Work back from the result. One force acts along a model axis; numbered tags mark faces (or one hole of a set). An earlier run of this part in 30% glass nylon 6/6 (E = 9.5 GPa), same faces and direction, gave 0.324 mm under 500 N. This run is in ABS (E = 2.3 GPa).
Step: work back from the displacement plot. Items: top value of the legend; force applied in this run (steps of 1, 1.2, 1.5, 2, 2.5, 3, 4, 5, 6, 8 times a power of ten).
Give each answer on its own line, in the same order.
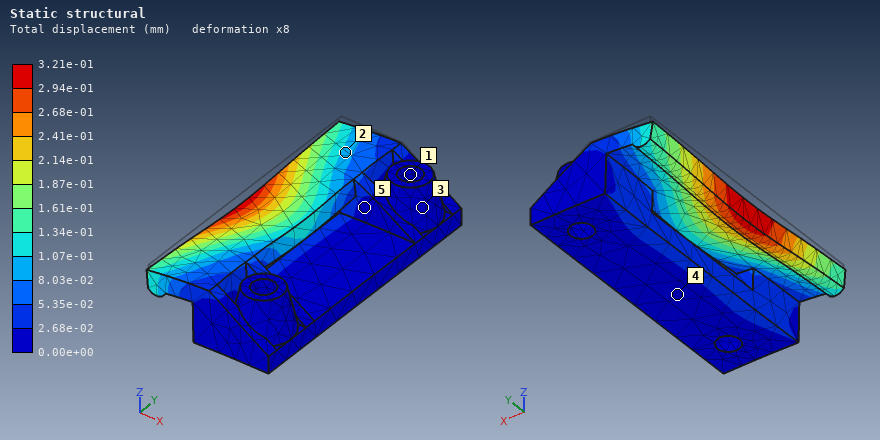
3.21e-01 mm
120 N
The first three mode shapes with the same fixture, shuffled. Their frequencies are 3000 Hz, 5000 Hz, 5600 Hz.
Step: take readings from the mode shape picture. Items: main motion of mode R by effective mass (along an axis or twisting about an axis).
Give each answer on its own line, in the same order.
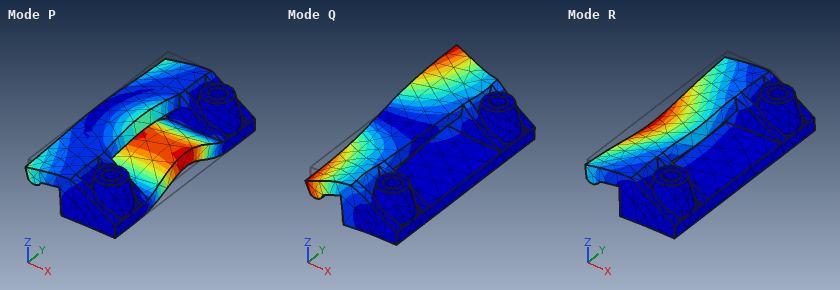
along Z
